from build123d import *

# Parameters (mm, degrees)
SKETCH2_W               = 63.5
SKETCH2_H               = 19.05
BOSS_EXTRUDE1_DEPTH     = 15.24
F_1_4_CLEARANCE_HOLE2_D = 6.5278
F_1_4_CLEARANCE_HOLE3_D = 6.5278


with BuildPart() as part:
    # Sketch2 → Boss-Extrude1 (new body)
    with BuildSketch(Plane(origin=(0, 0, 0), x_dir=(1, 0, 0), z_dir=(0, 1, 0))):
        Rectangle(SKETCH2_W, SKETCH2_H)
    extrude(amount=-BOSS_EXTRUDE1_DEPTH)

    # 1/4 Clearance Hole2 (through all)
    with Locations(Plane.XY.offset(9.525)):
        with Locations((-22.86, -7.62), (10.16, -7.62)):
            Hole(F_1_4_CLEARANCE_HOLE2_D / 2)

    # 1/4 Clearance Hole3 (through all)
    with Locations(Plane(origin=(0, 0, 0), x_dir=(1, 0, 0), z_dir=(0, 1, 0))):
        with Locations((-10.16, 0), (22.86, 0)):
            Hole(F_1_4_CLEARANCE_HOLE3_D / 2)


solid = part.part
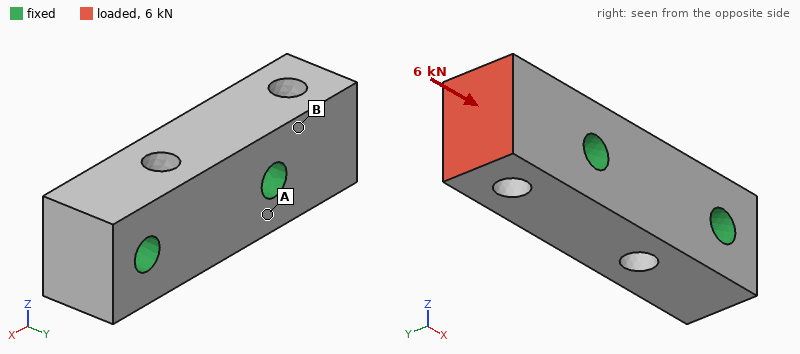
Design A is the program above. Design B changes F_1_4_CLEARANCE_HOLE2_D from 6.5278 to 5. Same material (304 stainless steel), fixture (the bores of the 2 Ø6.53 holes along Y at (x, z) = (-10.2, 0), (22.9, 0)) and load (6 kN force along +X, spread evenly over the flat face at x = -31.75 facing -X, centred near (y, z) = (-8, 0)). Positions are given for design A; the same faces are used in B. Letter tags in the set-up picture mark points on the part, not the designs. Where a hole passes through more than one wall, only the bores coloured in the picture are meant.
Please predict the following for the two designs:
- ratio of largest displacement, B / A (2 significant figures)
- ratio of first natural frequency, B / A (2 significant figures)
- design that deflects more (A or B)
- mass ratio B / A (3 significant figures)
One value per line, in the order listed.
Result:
0.83
1.0
A
1.03
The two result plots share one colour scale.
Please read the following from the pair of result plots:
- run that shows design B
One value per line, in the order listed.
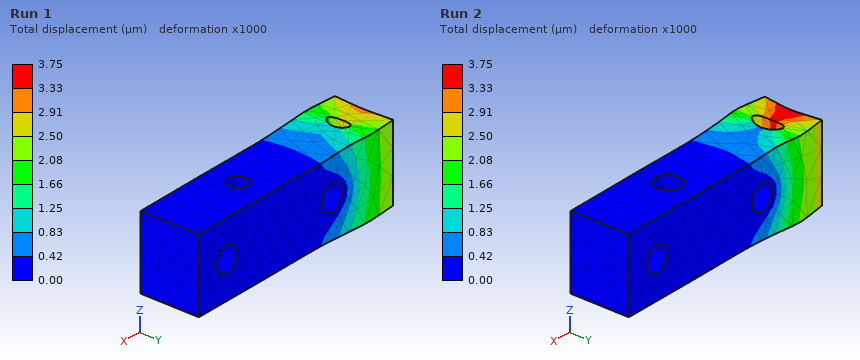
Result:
Run 1
